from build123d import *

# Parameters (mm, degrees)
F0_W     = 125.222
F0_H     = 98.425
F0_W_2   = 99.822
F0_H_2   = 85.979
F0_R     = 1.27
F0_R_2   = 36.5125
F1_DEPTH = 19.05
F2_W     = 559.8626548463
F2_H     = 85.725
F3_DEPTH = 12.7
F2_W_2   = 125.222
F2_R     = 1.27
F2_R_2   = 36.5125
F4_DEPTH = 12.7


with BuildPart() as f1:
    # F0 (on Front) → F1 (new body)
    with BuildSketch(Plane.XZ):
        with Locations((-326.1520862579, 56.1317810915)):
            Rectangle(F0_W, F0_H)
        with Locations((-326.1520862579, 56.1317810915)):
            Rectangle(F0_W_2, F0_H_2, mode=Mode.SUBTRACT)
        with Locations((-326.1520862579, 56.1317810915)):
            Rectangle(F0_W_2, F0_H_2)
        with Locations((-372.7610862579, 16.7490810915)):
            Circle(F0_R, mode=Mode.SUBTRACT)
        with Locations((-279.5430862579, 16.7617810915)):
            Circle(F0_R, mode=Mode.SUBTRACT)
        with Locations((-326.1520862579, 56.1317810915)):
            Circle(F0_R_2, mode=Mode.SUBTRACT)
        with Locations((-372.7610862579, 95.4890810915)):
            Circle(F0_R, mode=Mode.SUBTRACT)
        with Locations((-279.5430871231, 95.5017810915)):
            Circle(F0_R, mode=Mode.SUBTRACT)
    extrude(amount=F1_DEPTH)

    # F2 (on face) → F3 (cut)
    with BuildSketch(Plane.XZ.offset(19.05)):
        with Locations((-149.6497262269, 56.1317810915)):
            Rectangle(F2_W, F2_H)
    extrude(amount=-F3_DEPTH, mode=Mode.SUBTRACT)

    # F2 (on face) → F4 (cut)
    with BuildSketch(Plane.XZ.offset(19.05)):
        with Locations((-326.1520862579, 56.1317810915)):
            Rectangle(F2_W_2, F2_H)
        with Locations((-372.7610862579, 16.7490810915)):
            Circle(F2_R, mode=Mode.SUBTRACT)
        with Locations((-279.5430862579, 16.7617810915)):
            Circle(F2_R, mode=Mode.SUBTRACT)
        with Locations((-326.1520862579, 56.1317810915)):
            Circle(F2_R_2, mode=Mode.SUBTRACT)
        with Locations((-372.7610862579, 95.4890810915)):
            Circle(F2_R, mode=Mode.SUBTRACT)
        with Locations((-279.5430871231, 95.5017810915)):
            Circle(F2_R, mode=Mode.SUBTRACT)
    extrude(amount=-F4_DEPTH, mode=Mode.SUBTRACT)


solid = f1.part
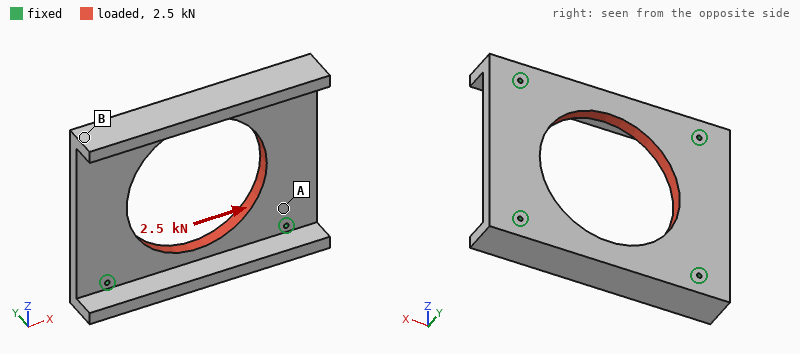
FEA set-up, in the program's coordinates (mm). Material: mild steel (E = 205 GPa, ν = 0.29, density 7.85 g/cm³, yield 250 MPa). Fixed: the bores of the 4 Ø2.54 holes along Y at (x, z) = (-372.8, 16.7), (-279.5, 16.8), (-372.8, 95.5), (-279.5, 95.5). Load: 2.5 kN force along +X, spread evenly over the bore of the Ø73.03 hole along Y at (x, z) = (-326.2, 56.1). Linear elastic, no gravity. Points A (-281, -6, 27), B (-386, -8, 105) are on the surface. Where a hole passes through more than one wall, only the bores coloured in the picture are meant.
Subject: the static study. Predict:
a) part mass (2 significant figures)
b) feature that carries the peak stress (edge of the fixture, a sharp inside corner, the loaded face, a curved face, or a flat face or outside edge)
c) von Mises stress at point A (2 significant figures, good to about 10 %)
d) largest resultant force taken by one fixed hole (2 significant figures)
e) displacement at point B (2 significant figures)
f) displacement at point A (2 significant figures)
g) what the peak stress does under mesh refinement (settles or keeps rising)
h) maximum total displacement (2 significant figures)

560 g
edge of the fixture
2.6 MPa
630 N
0.46 µm
0.71 µm
keeps rising
1.7 µm
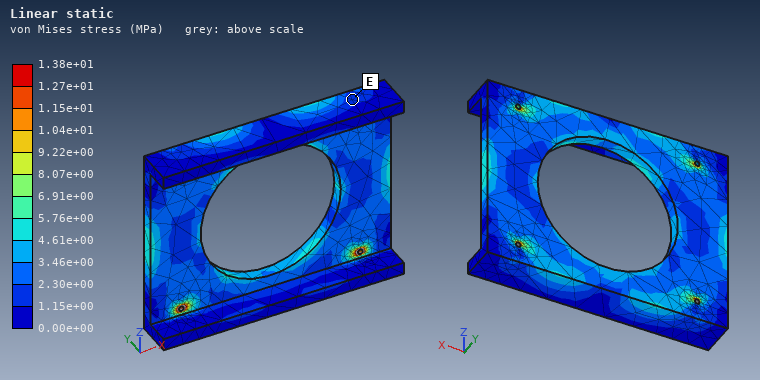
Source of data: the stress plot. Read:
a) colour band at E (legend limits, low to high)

1.15e+00 to 2.30e+00 MPa
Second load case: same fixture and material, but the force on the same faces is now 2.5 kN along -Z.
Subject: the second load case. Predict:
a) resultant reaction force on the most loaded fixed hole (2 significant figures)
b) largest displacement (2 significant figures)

630 N
3.0 µm
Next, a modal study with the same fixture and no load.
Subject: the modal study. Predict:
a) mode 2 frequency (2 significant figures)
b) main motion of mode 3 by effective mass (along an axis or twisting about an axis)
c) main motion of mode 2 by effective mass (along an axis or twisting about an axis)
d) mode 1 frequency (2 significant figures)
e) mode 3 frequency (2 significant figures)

4500 Hz
along Y
twisting about Z
4000 Hz
5200 Hz
